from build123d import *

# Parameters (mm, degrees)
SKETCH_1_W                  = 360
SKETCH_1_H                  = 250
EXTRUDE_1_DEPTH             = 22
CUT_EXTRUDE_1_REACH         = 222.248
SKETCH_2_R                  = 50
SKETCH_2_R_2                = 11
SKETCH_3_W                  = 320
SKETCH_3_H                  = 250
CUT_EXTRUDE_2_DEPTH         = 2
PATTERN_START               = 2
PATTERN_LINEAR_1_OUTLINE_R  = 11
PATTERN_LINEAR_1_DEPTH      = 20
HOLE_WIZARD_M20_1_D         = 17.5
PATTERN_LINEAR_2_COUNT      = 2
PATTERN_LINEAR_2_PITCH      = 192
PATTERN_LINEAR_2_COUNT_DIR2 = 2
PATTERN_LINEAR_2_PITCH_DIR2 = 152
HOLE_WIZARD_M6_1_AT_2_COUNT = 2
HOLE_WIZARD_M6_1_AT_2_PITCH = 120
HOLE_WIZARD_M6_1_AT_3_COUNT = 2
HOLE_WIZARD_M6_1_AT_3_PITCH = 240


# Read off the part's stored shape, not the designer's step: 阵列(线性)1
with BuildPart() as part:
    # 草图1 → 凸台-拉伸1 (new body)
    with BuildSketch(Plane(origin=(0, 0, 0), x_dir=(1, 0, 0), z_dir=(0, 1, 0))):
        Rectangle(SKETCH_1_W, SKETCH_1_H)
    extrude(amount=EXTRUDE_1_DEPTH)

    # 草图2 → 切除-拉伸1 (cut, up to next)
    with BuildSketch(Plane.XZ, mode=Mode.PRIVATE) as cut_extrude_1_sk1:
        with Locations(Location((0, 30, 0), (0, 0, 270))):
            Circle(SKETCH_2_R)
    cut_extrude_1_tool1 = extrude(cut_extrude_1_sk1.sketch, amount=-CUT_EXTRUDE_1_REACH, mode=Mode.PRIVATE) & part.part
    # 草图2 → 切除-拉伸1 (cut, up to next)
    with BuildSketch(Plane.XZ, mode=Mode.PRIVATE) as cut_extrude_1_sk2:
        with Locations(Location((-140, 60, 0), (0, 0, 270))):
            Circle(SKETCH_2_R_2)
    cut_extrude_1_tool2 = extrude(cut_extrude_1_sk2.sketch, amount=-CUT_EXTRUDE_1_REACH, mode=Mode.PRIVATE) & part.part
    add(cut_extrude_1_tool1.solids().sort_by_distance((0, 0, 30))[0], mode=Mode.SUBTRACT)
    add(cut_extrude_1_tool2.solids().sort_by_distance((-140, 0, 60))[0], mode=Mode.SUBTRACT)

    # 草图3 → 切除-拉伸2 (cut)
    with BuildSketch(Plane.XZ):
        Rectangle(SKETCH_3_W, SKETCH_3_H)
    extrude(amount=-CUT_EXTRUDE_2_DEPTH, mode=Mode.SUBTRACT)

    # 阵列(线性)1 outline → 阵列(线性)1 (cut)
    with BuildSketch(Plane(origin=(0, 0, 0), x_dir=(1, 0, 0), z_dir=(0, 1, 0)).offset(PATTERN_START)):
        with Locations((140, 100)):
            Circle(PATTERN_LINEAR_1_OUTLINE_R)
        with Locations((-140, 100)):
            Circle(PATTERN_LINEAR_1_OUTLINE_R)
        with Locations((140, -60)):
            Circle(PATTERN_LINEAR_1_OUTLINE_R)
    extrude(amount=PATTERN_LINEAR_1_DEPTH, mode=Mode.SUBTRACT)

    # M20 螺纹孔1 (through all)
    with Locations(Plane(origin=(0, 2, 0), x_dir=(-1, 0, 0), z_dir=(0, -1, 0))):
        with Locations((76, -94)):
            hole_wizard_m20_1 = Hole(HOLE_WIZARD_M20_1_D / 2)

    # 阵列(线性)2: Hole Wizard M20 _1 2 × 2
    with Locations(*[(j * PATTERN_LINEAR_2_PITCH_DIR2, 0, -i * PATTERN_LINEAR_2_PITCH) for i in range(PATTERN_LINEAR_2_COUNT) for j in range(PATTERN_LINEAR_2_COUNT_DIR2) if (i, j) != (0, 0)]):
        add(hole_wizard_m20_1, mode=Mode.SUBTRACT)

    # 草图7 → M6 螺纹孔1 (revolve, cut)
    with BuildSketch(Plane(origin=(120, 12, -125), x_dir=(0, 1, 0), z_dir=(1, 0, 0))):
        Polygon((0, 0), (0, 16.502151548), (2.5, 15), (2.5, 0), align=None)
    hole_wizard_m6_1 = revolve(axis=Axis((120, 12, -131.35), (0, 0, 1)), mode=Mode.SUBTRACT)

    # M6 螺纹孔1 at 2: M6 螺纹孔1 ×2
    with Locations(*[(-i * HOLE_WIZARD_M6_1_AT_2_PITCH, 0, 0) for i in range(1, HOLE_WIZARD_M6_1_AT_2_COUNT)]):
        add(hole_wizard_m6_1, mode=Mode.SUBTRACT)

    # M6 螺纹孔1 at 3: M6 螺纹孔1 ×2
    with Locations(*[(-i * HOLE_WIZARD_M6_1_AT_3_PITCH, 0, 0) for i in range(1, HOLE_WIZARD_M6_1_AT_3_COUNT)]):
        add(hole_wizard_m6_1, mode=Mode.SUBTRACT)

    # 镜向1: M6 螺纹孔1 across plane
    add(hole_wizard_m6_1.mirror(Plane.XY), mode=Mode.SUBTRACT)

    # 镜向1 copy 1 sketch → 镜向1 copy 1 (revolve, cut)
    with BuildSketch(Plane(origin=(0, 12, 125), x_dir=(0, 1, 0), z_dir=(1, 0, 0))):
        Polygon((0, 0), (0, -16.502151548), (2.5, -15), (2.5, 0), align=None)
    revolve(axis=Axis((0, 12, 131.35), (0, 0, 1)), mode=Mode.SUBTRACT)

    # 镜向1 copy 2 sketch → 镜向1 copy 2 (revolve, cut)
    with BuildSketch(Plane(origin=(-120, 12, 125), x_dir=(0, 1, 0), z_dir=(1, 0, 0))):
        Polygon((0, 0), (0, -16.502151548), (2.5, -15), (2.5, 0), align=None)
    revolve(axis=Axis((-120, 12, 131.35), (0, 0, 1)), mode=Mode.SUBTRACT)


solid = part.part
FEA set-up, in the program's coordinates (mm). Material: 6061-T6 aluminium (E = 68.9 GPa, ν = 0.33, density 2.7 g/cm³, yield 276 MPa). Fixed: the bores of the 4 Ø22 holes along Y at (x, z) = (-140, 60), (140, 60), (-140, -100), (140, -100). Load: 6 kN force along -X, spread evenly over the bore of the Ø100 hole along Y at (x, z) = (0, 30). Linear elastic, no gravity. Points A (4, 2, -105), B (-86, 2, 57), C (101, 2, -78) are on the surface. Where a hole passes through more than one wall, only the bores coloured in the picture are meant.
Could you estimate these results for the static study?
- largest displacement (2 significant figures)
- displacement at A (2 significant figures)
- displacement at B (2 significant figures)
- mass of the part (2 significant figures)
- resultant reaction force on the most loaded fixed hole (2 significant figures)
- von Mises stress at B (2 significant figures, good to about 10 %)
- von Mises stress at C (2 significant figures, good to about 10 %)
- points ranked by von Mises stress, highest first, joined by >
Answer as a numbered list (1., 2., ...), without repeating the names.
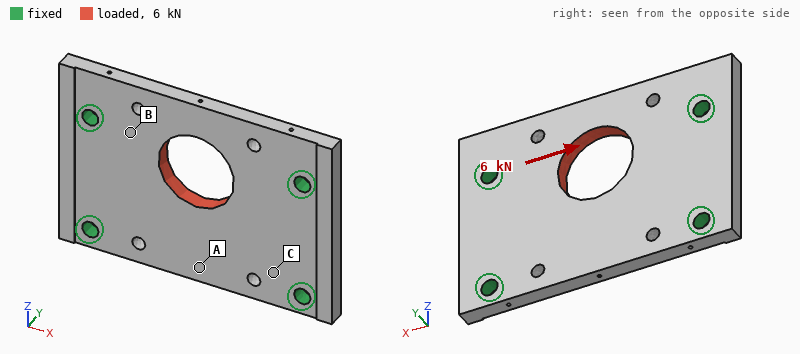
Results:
1. 2.4 µm
2. 0.56 µm
3. 1.1 µm
4. 4.4 kg
5. 2.1 kN
6. 1.3 MPa
7. 0.75 MPa
8. B > C > A
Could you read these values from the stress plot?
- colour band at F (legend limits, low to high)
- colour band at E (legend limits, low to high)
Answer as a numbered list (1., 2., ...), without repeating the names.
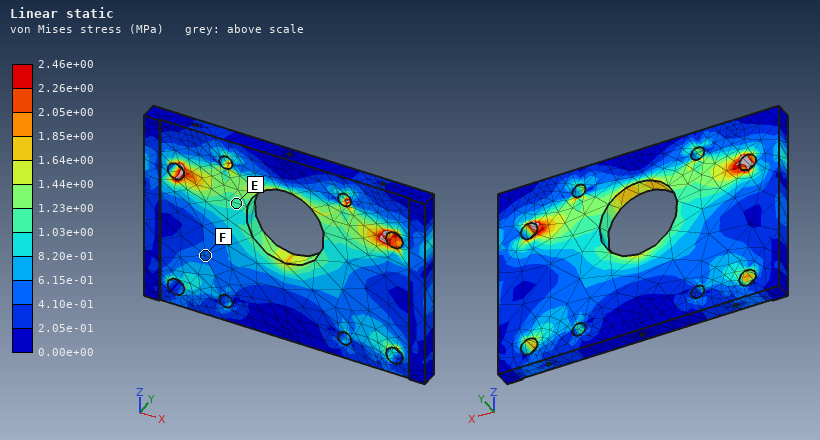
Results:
1. 4.10e-01 to 6.15e-01 MPa
2. 1.03e+00 to 1.23e+00 MPa
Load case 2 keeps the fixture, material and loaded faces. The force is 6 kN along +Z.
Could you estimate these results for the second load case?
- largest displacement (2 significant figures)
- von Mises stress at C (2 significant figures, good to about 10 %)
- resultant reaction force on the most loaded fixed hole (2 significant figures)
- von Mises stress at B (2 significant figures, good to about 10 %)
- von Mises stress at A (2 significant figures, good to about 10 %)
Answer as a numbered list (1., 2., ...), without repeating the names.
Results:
1. 5.9 µm
2. 1.3 MPa
3. 1.8 kN
4. 1.3 MPa
5. 0.55 MPa
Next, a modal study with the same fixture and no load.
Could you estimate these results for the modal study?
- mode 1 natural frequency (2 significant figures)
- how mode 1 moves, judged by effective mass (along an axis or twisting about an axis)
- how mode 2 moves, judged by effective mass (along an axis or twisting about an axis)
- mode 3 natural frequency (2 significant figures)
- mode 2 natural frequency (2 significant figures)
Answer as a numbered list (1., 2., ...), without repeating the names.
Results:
1. 1300 Hz
2. along Y
3. twisting about X
4. 2500 Hz
5. 1500 Hz
